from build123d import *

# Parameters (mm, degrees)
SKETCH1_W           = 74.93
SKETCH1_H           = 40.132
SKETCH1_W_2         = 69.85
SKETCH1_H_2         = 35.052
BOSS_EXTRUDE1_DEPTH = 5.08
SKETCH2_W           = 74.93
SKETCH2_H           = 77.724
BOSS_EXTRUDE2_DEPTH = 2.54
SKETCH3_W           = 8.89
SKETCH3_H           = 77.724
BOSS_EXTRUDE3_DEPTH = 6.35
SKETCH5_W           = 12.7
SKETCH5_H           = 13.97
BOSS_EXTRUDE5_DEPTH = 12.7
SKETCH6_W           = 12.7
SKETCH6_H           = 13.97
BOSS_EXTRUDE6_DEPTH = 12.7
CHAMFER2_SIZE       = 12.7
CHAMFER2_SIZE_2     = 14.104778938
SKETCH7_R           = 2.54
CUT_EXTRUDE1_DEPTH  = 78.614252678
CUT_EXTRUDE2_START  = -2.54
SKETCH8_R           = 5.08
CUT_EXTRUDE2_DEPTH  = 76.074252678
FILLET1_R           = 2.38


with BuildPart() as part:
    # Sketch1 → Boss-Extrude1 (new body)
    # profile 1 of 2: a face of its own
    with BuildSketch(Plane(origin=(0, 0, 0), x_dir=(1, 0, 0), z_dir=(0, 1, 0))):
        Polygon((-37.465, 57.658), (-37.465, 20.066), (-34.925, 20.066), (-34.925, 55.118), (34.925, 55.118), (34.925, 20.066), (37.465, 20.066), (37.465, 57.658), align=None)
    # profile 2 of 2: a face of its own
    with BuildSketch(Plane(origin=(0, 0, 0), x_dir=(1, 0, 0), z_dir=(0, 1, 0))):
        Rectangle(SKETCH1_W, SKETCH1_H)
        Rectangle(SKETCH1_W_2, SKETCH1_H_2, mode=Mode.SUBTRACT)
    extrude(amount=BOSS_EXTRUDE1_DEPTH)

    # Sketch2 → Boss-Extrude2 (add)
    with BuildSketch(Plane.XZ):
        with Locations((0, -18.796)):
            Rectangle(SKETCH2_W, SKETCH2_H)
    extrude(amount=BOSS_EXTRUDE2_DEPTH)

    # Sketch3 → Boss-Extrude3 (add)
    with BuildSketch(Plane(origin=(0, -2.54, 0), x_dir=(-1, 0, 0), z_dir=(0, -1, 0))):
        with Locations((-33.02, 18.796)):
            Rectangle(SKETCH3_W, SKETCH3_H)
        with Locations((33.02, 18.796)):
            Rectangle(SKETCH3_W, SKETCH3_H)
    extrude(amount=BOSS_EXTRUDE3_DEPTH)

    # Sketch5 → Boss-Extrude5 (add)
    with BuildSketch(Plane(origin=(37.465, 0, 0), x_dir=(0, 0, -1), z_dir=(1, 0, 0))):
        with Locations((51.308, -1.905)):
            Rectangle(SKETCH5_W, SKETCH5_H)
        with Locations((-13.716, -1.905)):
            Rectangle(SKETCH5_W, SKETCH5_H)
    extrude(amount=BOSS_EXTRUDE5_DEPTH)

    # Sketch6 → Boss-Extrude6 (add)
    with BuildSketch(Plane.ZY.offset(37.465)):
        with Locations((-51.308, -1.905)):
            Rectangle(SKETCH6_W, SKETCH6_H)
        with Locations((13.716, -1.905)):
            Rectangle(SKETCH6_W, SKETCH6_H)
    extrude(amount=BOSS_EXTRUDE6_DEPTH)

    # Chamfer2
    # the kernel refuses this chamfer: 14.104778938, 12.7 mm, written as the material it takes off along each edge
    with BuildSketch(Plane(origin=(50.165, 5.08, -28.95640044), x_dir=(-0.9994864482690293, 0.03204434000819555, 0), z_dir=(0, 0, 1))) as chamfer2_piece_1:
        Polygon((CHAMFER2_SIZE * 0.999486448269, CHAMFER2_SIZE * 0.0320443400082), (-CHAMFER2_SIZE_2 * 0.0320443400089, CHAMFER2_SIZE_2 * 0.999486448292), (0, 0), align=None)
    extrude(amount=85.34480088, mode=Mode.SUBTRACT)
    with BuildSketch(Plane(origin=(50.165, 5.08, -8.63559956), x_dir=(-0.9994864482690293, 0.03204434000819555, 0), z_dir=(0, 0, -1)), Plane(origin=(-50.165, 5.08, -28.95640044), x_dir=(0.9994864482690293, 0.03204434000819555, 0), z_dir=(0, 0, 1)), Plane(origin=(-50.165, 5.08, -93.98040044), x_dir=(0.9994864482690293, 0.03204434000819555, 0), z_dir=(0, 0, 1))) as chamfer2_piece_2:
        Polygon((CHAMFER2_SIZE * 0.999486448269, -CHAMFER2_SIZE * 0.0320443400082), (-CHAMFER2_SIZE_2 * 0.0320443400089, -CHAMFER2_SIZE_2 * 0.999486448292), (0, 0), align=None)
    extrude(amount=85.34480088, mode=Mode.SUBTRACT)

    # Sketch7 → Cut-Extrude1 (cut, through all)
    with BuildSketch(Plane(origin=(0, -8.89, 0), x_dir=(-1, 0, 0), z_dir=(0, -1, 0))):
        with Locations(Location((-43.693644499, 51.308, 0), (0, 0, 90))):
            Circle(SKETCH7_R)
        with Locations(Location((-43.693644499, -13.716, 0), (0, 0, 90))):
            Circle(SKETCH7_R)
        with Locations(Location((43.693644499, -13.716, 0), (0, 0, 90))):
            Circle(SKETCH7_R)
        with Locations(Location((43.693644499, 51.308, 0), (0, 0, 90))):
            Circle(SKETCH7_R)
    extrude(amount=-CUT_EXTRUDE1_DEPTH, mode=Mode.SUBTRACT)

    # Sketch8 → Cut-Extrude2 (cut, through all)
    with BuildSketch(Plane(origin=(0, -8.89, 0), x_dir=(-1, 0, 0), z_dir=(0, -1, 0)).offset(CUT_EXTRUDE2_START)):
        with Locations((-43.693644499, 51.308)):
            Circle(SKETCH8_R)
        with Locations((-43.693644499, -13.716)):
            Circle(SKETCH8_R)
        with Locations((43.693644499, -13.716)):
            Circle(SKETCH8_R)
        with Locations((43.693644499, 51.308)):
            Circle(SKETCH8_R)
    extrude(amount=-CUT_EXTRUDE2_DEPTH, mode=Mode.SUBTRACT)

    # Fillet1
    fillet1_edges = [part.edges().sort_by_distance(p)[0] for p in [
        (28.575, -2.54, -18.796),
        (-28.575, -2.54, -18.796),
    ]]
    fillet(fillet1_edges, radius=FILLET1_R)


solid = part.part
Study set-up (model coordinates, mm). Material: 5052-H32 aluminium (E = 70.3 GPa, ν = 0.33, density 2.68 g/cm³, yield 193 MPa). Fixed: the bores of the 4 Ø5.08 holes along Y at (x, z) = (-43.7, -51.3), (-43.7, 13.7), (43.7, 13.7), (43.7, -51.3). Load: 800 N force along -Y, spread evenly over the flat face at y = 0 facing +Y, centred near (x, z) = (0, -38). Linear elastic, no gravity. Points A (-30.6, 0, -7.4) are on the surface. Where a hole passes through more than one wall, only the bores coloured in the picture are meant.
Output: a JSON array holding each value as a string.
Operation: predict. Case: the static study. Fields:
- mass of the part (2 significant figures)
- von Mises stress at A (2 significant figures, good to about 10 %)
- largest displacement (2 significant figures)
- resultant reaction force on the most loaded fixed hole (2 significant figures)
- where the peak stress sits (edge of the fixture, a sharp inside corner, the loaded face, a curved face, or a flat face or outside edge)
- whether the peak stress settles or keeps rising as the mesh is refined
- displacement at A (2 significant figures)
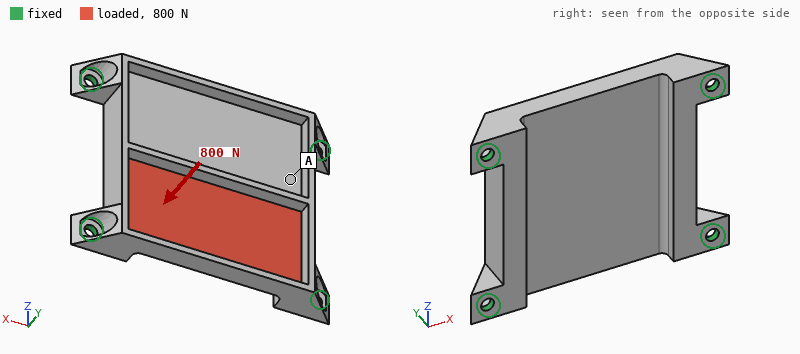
["84 g", "5.1 MPa", "64 µm", "760 N", "edge of the fixture", "keeps rising", "11 µm"]
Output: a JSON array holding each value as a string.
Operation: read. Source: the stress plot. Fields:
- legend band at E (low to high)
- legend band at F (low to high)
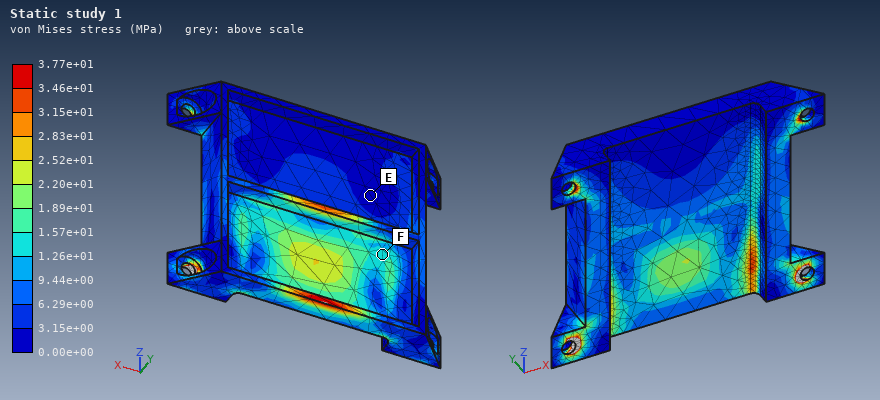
["0.00e+00 to 3.15e+00 MPa", "1.26e+01 to 1.57e+01 MPa"]
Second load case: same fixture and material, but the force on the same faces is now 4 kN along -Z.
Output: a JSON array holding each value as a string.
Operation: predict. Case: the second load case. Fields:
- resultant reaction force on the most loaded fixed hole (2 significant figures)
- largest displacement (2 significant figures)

["1.2 kN", "39 µm"]
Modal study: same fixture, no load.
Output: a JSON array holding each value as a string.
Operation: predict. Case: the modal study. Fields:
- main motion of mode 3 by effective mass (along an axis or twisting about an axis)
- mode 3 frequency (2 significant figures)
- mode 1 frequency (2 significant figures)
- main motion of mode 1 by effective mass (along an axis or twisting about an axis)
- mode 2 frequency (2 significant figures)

["twisting about X", "5500 Hz", "3900 Hz", "along Y", "5100 Hz"]
